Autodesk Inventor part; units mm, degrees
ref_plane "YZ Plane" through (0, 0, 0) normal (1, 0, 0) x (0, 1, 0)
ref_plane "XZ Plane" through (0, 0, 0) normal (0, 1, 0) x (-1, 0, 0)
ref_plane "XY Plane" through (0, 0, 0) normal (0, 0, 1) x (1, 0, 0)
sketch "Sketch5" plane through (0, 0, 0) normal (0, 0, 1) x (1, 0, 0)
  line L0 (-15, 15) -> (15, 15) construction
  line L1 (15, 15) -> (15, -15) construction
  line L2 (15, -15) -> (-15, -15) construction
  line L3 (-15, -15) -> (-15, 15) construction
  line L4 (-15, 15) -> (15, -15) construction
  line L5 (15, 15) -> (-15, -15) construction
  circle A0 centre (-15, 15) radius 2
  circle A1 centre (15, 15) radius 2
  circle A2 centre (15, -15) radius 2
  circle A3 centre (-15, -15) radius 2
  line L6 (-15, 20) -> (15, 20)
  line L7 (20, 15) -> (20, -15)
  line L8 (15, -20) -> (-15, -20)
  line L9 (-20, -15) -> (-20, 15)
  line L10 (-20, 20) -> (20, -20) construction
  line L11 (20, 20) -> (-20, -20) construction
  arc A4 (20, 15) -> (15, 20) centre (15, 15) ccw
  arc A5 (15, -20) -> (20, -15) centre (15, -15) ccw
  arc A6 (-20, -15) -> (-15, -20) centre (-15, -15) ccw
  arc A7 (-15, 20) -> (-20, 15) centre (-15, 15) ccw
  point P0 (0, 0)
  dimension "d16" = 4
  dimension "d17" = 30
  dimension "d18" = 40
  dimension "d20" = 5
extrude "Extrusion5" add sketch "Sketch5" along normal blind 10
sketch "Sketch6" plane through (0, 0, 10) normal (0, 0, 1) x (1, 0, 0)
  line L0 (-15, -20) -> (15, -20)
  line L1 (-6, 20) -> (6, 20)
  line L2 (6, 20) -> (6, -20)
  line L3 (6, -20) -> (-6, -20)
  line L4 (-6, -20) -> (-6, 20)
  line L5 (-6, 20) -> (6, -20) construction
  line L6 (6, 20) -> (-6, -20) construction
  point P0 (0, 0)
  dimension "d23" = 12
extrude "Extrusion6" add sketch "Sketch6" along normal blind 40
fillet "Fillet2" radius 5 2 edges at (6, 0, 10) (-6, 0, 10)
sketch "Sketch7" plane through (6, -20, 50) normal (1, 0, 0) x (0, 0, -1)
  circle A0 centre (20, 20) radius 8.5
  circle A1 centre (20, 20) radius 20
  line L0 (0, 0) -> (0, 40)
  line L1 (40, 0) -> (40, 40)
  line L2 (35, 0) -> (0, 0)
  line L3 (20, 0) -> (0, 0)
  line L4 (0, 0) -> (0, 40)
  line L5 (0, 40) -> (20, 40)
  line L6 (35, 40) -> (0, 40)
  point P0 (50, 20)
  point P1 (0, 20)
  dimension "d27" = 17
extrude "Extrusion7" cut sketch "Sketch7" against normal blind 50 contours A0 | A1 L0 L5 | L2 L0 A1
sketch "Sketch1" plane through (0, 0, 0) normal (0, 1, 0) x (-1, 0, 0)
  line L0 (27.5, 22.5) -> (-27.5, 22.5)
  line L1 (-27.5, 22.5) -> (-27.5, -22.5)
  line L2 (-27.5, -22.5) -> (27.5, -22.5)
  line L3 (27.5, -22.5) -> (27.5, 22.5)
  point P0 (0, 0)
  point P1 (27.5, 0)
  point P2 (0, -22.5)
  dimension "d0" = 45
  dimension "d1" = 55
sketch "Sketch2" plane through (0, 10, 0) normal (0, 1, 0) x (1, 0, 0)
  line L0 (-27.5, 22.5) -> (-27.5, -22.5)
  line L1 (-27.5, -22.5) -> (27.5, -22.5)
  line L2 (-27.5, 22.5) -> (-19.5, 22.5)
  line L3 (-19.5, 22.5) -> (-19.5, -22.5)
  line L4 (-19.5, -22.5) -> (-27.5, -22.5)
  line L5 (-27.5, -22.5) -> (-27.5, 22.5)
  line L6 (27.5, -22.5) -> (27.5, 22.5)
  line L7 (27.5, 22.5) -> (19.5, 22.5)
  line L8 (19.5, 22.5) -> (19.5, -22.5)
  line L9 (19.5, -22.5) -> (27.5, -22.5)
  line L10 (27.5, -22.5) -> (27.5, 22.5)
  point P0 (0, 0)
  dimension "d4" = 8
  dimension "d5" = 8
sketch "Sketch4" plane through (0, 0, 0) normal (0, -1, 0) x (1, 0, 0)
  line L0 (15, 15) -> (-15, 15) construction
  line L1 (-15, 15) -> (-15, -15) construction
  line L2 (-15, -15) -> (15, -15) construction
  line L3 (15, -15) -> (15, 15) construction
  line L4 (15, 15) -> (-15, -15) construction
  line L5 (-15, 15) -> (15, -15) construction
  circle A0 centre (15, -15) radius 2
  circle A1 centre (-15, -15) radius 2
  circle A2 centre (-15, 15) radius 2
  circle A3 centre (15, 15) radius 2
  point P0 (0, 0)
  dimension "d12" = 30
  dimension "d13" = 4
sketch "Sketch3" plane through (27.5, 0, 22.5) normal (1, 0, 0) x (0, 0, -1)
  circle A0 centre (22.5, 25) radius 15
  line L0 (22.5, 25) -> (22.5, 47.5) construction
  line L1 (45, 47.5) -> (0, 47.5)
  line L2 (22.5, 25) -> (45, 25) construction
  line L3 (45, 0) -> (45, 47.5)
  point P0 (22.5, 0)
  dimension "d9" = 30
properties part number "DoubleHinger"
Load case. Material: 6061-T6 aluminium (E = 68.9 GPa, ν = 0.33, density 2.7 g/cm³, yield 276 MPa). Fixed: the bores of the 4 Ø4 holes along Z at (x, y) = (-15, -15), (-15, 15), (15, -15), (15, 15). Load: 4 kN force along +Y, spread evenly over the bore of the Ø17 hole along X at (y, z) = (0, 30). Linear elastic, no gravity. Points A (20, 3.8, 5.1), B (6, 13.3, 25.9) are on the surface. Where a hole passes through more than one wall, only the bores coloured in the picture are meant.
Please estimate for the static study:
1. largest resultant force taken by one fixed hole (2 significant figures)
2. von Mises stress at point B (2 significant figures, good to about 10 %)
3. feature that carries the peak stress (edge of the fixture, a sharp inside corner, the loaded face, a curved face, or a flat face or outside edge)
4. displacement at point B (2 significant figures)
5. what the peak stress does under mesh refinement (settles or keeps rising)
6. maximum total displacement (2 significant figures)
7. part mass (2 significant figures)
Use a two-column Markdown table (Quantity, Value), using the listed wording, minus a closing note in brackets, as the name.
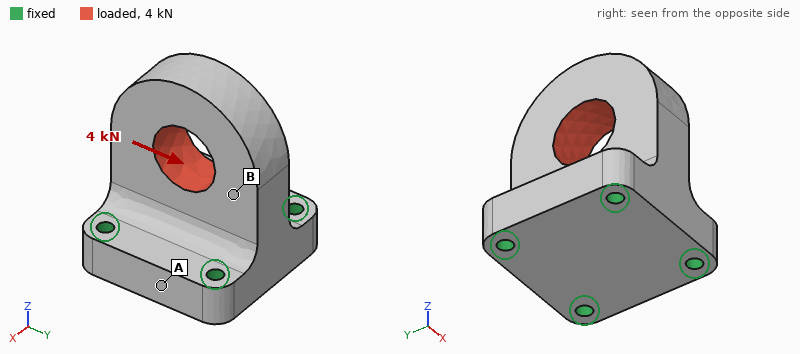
| Quantity | Value |
|---|---|
| largest resultant force taken by one fixed hole | 2.0 kN |
| von Mises stress at point B | 22 MPa |
| feature that carries the peak stress | edge of the fixture |
| displacement at point B | 23 µm |
| what the peak stress does under mesh refinement | keeps rising |
| maximum total displacement | 45 µm |
| part mass | 81 g |
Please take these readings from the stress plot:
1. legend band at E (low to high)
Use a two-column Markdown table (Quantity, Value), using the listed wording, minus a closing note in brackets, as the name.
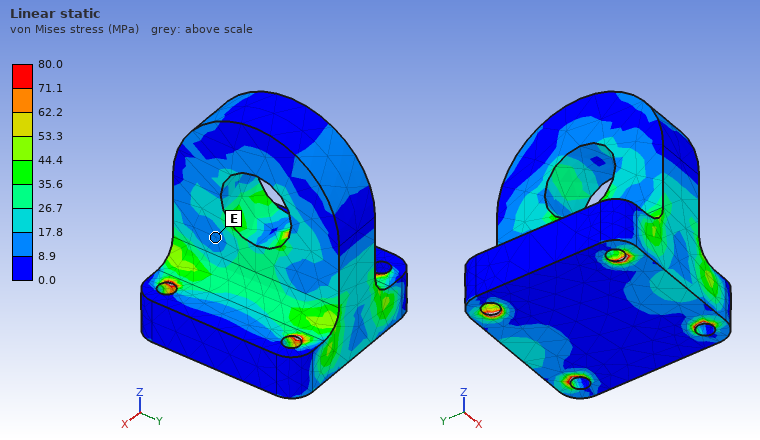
| Quantity | Value |
|---|---|
| legend band at E | 8.9 to 17.8 MPa |
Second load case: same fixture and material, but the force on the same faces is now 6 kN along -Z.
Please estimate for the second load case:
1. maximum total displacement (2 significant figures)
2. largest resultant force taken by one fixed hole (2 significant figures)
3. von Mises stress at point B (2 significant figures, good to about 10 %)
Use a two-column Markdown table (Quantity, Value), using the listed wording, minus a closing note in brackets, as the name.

| Quantity | Value |
|---|---|
| maximum total displacement | 15 µm |
| largest resultant force taken by one fixed hole | 1.6 kN |
| von Mises stress at point B | 15 MPa |
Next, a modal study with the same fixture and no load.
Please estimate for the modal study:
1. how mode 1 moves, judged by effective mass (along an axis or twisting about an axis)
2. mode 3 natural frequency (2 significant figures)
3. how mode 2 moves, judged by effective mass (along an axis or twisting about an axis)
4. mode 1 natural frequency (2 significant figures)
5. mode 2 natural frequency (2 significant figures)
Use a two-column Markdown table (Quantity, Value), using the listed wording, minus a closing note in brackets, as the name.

| Quantity | Value |
|---|---|
| how mode 1 moves, judged by effective mass | along X |
| mode 3 natural frequency | 13 kHz |
| how mode 2 moves, judged by effective mass | along Y |
| mode 1 natural frequency | 6000 Hz |
| mode 2 natural frequency | 9100 Hz |
